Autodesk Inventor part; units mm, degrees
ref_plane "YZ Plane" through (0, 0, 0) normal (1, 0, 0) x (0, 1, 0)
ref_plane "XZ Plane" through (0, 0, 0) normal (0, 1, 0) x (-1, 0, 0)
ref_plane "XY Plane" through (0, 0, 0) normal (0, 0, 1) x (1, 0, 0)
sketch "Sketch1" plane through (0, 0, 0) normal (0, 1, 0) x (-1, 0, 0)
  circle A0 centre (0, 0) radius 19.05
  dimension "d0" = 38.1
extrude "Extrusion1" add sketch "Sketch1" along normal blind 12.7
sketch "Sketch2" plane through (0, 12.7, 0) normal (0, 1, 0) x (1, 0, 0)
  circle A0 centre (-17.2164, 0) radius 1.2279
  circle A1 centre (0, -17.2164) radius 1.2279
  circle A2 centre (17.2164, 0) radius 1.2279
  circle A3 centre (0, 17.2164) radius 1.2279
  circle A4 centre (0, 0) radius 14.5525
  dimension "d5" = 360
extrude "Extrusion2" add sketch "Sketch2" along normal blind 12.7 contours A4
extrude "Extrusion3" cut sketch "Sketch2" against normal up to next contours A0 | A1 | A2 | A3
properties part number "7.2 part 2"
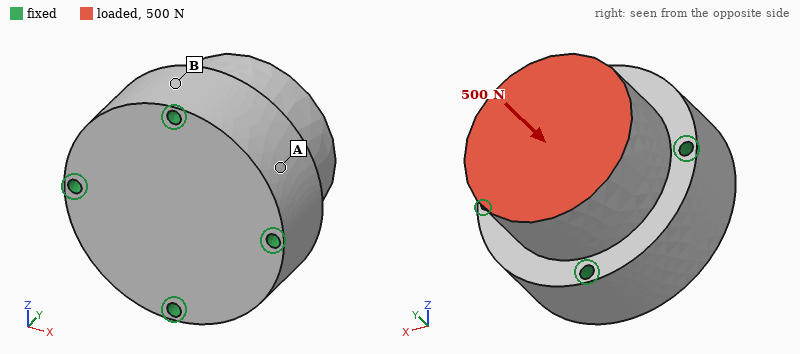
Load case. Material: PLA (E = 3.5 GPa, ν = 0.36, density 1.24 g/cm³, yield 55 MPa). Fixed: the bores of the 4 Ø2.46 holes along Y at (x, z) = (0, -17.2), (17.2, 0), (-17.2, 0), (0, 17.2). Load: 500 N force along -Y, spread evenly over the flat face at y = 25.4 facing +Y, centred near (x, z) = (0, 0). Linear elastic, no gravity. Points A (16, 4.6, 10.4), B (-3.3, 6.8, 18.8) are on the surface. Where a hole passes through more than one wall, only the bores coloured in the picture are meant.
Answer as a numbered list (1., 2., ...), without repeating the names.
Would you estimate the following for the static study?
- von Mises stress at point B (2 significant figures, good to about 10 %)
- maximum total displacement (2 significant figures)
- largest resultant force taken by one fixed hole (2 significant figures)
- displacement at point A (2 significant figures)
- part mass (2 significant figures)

1. 1.0 MPa
2. 7.7 µm
3. 130 N
4. 3.8 µm
5. 28 g
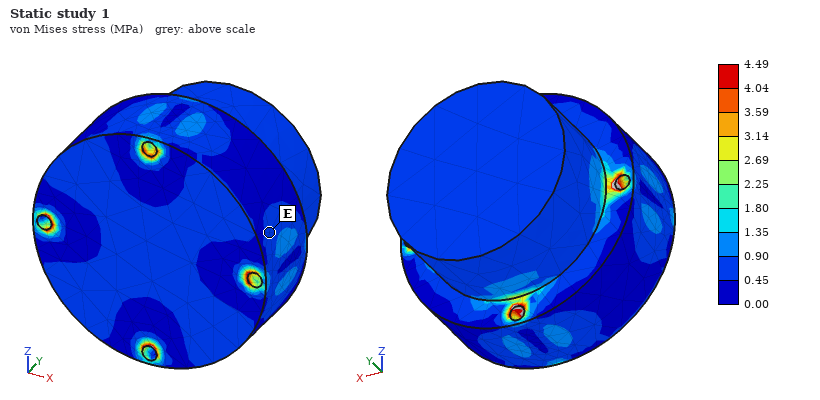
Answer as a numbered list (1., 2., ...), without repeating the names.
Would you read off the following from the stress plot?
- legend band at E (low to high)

1. 0.45 to 0.90 MPa
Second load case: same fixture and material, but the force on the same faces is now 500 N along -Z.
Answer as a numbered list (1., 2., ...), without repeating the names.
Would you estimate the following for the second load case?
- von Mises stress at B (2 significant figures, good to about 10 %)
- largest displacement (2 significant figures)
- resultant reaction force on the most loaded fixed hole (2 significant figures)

1. 2.6 MPa
2. 30 µm
3. 300 N
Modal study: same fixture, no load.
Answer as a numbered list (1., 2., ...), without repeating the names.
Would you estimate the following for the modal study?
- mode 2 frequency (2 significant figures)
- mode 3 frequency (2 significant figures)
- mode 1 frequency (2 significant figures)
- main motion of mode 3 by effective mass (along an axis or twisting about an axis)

1. 8900 Hz
2. 10 kHz
3. 8900 Hz
4. along Y
